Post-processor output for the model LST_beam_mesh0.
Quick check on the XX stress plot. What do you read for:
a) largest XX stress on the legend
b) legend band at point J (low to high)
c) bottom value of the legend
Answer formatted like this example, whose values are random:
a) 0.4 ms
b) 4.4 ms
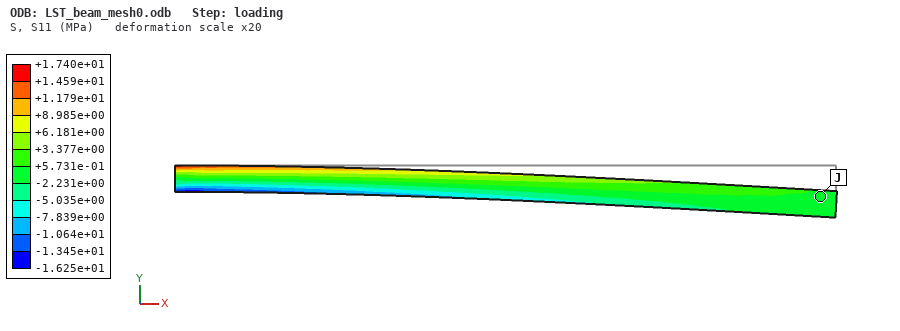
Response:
a) +1.740e+01 MPa
b) -2.231e+00 to +5.731e-01 MPa
c) -1.625e+01 MPa
